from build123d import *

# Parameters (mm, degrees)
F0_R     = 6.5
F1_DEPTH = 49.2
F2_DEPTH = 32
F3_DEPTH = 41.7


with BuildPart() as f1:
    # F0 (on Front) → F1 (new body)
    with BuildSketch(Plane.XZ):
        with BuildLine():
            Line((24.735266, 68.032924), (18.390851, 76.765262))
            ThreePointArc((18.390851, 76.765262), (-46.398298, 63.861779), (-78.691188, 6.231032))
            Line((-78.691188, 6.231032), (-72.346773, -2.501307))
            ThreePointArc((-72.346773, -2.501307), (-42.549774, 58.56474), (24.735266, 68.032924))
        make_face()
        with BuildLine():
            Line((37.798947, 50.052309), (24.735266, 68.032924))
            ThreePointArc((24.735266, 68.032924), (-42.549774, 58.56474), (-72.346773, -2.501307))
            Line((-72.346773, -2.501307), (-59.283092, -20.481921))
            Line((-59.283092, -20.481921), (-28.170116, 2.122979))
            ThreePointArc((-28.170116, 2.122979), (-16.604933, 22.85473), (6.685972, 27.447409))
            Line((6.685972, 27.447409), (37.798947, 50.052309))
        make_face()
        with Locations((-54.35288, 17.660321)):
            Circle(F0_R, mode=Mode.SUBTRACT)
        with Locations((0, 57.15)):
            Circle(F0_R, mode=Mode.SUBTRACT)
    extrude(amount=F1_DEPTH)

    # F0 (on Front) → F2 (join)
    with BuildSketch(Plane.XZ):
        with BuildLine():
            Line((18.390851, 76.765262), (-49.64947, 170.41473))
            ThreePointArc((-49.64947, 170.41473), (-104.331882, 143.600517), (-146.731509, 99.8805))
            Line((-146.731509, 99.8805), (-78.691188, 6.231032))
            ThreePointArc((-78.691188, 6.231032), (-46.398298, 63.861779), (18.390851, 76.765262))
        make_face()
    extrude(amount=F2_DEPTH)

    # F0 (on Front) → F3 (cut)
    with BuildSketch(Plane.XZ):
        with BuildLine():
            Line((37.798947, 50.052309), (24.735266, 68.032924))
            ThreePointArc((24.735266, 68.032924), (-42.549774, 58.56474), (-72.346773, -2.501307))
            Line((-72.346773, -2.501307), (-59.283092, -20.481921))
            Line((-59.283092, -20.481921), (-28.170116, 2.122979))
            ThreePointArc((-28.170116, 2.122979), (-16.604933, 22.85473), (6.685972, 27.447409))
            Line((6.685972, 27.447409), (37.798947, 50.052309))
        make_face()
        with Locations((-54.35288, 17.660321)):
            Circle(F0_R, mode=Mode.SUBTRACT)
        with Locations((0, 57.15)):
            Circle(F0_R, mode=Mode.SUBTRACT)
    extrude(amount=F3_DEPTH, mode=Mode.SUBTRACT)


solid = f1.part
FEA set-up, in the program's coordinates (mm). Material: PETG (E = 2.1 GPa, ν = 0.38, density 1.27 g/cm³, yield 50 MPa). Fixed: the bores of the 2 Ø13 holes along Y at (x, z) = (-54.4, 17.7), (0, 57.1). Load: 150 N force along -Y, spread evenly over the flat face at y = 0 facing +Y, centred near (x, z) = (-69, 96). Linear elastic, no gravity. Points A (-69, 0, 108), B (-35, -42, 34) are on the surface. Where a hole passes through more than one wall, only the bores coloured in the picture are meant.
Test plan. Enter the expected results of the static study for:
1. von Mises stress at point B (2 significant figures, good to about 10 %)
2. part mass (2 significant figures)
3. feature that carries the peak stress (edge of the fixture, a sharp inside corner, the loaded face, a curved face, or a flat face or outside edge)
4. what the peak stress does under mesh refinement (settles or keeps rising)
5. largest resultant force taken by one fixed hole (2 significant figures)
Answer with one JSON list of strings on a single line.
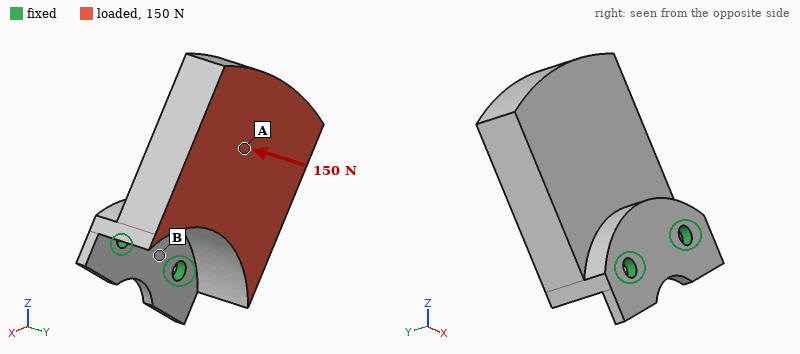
["2.5 MPa", "610 g", "edge of the fixture", "keeps rising", "97 N"]
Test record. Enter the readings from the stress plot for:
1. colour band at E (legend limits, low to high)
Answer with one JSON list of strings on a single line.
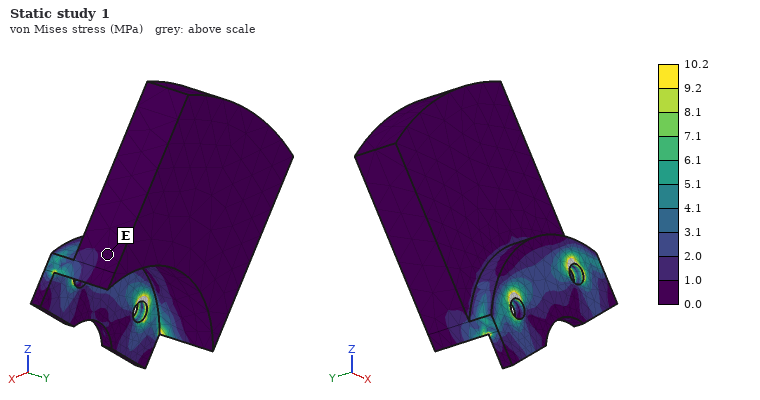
["0.0 to 1.0 MPa"]
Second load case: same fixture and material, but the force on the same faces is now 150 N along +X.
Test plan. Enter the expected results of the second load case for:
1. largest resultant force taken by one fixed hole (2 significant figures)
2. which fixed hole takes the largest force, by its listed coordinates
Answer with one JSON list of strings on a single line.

["180 N", "(0, 57.1)"]
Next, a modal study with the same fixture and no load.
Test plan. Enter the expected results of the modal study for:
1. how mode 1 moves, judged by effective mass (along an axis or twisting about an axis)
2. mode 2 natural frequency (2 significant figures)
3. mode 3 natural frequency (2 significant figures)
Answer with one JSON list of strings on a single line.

["along Y", "320 Hz", "440 Hz"]
